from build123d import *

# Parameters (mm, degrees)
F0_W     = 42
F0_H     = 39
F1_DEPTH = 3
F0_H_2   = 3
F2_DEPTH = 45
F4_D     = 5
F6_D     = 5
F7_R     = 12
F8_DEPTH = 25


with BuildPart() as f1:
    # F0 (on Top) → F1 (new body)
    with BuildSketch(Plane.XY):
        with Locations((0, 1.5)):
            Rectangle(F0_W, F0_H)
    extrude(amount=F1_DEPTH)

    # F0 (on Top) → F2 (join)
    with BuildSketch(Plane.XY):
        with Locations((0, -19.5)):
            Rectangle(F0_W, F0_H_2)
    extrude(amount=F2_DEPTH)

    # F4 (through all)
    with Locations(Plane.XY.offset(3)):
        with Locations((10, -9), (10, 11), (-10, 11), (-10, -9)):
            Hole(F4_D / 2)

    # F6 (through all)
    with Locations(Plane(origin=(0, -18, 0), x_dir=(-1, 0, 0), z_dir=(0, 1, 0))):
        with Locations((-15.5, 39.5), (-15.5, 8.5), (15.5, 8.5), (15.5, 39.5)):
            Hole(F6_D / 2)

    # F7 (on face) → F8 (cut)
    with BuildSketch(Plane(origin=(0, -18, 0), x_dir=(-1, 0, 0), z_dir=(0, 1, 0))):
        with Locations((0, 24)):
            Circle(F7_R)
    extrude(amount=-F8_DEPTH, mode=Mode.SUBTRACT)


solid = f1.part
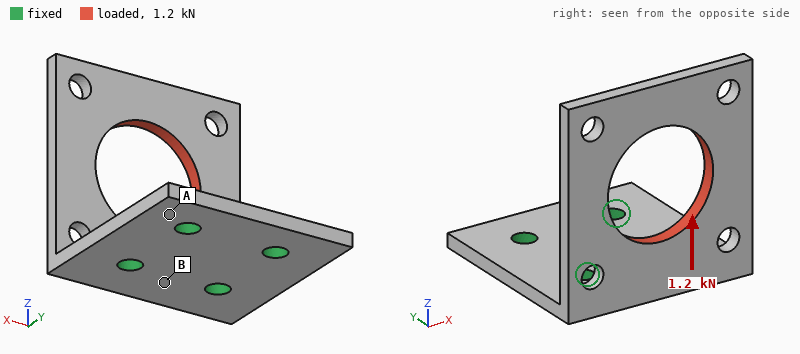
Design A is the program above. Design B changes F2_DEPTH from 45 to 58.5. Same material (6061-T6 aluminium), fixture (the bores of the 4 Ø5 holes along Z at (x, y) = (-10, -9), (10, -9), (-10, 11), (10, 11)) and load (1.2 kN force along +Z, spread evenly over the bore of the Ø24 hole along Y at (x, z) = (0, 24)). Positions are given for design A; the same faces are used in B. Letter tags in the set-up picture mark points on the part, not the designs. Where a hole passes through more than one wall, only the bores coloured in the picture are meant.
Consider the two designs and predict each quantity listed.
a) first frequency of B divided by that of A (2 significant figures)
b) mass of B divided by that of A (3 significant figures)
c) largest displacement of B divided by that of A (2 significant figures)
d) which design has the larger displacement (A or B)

0.55
1.19
1.3
B
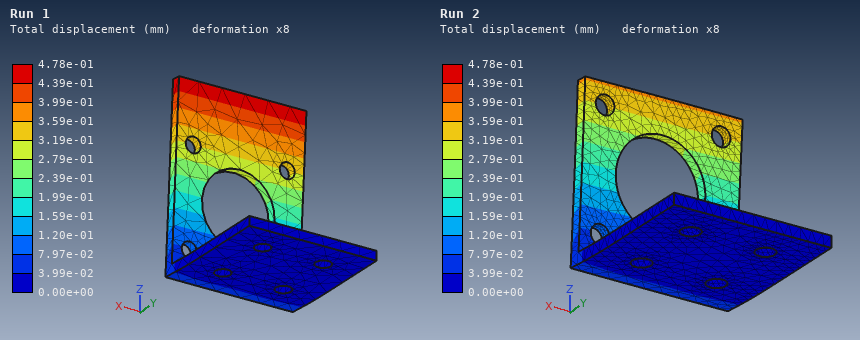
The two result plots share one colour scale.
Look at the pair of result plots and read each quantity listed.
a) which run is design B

Run 1
